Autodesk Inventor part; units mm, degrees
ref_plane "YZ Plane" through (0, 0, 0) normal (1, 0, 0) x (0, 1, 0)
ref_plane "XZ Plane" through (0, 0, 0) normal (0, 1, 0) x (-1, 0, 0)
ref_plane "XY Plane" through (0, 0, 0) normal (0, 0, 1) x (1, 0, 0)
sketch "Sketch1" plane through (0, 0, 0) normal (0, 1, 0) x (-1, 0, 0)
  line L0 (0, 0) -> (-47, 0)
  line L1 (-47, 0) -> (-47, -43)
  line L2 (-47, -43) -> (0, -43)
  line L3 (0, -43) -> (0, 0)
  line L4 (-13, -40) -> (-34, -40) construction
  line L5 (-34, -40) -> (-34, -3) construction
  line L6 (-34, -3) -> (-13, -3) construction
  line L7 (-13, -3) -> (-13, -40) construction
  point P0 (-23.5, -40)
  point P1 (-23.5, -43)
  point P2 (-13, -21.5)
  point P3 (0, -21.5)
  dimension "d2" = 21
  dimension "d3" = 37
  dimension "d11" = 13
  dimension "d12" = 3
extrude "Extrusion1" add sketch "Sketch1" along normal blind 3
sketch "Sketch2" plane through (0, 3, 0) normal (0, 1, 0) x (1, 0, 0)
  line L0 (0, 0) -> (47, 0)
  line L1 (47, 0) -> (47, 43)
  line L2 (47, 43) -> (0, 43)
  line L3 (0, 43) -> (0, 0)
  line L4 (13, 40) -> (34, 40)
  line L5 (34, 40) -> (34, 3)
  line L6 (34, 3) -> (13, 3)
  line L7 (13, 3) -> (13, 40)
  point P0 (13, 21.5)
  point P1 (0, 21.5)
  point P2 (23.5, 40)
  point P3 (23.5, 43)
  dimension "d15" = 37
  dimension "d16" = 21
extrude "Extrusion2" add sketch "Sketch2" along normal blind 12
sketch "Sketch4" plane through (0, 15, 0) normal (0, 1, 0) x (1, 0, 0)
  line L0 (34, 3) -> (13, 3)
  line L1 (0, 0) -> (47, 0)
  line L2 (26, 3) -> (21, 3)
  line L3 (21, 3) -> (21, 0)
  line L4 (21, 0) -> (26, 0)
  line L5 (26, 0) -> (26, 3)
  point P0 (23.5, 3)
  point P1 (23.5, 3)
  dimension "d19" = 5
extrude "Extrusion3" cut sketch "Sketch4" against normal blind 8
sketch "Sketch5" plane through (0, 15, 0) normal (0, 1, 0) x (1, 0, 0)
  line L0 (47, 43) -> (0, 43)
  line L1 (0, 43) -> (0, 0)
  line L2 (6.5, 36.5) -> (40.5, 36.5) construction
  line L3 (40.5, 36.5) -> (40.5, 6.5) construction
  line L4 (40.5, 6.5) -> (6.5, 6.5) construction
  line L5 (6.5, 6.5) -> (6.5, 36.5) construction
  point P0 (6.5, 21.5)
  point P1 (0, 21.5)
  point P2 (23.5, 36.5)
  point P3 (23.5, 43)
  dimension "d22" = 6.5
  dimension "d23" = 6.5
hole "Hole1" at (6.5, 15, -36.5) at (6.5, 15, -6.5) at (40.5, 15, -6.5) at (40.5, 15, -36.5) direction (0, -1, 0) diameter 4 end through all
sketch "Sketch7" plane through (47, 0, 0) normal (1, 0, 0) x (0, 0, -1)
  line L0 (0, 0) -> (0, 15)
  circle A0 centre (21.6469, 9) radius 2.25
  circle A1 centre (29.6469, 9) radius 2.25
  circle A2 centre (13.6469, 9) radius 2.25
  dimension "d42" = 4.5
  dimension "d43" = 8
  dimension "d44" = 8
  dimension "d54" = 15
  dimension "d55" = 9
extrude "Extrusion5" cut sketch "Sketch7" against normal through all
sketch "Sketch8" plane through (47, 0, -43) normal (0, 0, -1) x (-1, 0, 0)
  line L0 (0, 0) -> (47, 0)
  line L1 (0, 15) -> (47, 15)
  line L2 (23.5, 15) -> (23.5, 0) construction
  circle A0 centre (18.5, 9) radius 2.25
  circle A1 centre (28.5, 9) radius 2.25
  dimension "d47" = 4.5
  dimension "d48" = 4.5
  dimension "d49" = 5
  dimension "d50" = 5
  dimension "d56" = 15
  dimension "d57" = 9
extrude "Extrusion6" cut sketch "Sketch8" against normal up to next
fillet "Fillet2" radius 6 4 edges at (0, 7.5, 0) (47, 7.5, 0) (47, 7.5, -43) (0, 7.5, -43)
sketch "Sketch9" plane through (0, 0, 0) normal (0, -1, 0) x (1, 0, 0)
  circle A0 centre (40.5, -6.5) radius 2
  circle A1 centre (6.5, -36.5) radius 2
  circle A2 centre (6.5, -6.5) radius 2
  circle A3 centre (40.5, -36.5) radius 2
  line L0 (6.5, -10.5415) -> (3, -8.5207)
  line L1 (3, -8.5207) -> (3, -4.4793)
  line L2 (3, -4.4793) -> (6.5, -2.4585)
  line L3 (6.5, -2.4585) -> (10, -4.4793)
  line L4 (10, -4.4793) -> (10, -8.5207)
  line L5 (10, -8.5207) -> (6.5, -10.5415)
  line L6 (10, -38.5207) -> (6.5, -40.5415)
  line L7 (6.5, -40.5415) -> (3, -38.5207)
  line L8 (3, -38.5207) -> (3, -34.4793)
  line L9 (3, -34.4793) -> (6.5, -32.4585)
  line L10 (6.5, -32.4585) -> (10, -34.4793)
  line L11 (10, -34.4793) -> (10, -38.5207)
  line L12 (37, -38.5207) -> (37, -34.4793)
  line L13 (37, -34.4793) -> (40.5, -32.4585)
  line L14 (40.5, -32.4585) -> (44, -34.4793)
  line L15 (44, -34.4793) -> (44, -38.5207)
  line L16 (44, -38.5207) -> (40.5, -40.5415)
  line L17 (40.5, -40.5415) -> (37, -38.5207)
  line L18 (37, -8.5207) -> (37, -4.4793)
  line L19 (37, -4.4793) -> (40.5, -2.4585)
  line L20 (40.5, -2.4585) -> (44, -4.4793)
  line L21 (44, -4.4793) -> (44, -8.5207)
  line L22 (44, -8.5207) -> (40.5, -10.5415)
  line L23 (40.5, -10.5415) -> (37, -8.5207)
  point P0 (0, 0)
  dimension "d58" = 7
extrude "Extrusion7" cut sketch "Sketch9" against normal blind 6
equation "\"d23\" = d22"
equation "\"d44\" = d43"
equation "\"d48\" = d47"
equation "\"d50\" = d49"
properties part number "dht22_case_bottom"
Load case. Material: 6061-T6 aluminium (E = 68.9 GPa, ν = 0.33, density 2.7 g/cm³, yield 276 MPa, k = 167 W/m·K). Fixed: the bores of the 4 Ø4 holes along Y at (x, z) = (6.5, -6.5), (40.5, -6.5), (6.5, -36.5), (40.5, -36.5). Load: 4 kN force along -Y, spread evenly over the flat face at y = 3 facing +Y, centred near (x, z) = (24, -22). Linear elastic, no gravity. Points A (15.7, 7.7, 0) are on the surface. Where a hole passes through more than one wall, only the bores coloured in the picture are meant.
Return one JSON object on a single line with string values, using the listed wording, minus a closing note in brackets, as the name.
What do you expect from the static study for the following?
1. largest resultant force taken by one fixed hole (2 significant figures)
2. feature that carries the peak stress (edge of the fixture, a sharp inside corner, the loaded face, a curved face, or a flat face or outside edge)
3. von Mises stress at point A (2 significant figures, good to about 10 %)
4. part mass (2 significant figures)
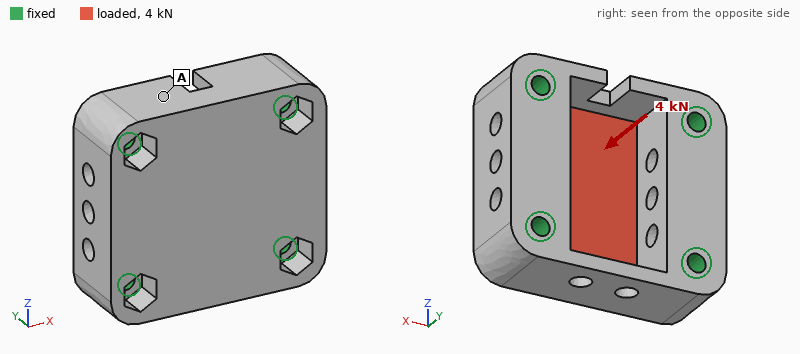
{"largest resultant force taken by one fixed hole": "1.3 kN", "feature that carries the peak stress": "a flat face or outside edge", "von Mises stress at point A": "8.9 MPa", "part mass": "48 g"}
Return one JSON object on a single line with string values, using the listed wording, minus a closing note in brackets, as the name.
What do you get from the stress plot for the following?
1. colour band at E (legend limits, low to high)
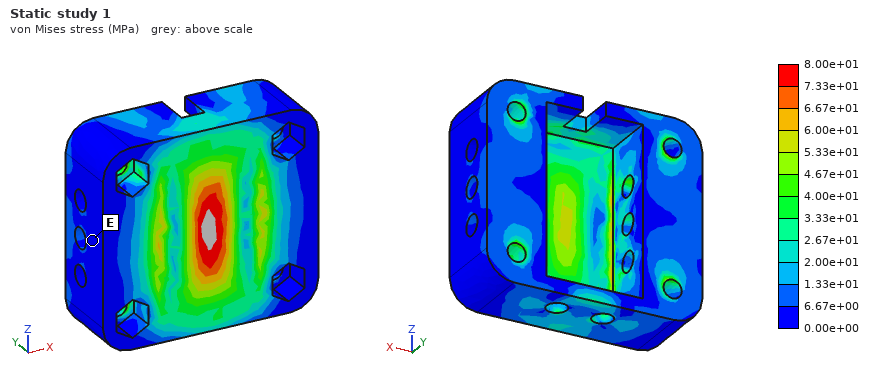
{"colour band at E": "0.00e+00 to 6.67e+00 MPa"}
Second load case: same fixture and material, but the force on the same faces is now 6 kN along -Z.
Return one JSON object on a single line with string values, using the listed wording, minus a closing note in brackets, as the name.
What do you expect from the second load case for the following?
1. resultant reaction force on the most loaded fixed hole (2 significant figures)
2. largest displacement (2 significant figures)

{"resultant reaction force on the most loaded fixed hole": "1.6 kN", "largest displacement": "13 µm"}
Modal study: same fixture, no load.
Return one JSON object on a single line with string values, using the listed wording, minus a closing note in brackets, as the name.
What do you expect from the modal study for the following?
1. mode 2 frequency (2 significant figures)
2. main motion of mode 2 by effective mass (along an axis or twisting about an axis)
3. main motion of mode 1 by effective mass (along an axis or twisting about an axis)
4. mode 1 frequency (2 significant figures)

{"mode 2 frequency": "27 kHz", "main motion of mode 2 by effective mass": "along X", "main motion of mode 1 by effective mass": "along Y", "mode 1 frequency": "24 kHz"}
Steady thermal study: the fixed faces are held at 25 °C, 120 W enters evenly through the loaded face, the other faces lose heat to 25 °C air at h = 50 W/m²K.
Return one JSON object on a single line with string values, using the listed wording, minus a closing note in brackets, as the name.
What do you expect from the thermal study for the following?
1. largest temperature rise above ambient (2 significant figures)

{"largest temperature rise above ambient": "33 K"}
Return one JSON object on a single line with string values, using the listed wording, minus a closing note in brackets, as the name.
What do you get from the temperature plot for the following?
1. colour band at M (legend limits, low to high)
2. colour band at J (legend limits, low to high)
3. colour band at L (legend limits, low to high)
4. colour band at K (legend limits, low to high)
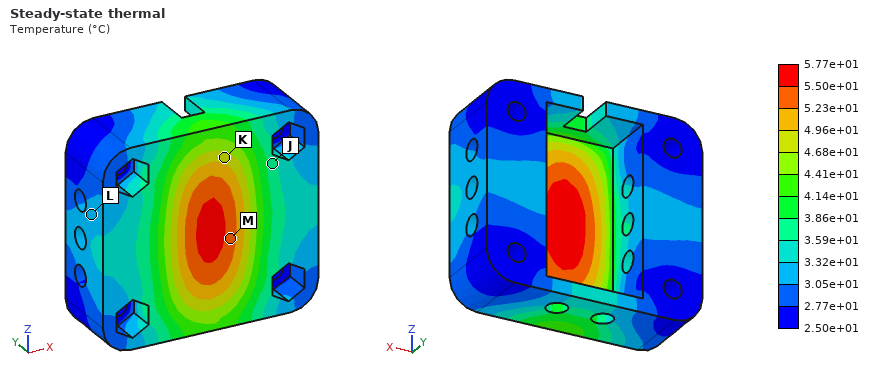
{"colour band at M": "5.23e+01 to 5.50e+01 °C", "colour band at J": "3.59e+01 to 3.86e+01 °C", "colour band at L": "3.05e+01 to 3.32e+01 °C", "colour band at K": "4.68e+01 to 4.96e+01 °C"}
